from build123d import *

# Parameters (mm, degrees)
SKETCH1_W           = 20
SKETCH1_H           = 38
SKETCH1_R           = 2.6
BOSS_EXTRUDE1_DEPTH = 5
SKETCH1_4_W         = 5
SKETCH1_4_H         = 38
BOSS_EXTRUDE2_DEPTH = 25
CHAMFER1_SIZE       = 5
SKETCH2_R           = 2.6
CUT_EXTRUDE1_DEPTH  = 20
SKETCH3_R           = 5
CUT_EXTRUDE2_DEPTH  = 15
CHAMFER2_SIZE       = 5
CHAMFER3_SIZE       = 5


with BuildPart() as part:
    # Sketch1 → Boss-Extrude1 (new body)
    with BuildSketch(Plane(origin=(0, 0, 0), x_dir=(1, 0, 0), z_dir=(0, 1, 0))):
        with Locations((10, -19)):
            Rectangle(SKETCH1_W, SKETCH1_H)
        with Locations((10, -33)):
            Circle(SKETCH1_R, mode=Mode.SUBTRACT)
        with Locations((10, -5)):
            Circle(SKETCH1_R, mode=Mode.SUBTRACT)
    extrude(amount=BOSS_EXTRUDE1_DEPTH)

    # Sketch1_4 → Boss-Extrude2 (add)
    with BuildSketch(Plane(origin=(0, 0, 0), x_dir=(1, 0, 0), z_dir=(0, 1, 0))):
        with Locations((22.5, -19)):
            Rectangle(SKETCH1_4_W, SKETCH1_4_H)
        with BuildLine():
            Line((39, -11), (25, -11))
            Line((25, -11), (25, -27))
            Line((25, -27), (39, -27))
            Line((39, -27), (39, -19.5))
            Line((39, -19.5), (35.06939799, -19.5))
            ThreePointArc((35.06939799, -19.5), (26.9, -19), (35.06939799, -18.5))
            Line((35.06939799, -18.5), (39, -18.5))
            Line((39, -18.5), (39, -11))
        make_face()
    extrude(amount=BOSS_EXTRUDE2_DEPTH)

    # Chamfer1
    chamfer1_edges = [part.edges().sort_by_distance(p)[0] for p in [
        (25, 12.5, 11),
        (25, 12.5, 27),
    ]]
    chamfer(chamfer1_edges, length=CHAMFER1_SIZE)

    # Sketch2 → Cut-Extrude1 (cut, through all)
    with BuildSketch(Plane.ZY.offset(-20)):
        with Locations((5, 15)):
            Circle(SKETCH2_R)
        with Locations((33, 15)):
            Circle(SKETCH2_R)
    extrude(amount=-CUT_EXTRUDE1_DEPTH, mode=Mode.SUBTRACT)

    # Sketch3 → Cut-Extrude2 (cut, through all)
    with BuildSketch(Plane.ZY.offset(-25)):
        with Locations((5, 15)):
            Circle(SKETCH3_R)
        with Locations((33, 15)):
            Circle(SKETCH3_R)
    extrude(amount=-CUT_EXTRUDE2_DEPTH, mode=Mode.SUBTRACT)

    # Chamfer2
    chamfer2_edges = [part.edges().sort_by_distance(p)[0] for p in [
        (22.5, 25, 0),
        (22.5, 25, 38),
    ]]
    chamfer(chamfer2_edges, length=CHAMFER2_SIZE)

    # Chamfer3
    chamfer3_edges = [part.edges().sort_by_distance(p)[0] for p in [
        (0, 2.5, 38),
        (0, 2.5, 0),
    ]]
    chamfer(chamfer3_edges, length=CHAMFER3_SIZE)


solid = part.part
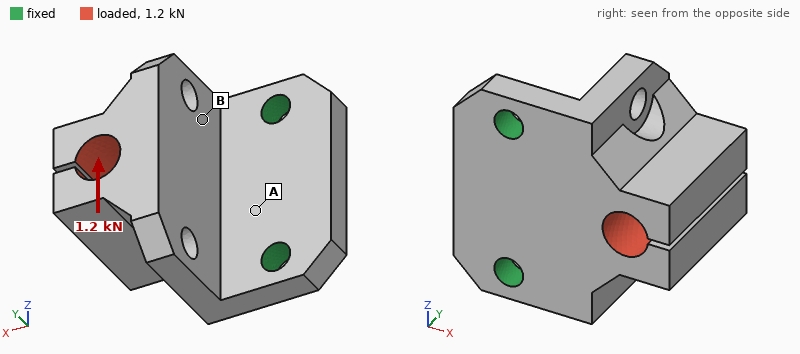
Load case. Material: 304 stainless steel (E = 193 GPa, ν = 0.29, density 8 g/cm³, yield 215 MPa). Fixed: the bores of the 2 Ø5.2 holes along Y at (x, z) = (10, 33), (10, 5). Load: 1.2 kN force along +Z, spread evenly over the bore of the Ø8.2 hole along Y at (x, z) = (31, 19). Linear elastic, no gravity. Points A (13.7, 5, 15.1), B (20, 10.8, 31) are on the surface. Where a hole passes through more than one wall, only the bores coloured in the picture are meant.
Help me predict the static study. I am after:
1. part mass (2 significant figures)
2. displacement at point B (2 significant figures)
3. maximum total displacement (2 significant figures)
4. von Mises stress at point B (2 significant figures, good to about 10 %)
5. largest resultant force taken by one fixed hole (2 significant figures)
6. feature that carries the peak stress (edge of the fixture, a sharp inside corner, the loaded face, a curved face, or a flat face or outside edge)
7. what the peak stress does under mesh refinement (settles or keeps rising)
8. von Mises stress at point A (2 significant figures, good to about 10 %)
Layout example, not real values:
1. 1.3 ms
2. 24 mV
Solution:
1. 100 g
2. 4.1 µm
3. 10 µm
4. 8.5 MPa
5. 1.1 kN
6. edge of the fixture
7. keeps rising
8. 18 MPa
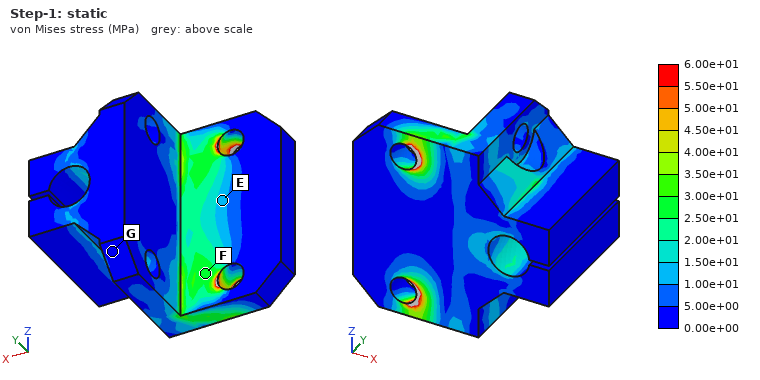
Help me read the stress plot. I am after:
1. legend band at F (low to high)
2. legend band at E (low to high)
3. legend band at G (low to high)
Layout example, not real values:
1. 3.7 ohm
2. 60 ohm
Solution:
1. 2.50e+01 to 3.00e+01 MPa
2. 1.00e+01 to 1.50e+01 MPa
3. 0.00e+00 to 5.00e+00 MPa
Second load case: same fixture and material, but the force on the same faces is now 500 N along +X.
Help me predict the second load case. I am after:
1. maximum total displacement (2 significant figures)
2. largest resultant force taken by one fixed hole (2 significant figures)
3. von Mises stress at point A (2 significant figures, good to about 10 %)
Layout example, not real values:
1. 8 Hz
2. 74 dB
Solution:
1. 27 µm
2. 260 N
3. 22 MPa
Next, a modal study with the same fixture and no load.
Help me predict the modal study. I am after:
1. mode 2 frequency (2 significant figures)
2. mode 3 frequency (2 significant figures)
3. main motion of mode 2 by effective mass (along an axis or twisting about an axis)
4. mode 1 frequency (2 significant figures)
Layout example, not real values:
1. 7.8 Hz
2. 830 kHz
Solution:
1. 7900 Hz
2. 11 kHz
3. along Z
4. 2600 Hz
